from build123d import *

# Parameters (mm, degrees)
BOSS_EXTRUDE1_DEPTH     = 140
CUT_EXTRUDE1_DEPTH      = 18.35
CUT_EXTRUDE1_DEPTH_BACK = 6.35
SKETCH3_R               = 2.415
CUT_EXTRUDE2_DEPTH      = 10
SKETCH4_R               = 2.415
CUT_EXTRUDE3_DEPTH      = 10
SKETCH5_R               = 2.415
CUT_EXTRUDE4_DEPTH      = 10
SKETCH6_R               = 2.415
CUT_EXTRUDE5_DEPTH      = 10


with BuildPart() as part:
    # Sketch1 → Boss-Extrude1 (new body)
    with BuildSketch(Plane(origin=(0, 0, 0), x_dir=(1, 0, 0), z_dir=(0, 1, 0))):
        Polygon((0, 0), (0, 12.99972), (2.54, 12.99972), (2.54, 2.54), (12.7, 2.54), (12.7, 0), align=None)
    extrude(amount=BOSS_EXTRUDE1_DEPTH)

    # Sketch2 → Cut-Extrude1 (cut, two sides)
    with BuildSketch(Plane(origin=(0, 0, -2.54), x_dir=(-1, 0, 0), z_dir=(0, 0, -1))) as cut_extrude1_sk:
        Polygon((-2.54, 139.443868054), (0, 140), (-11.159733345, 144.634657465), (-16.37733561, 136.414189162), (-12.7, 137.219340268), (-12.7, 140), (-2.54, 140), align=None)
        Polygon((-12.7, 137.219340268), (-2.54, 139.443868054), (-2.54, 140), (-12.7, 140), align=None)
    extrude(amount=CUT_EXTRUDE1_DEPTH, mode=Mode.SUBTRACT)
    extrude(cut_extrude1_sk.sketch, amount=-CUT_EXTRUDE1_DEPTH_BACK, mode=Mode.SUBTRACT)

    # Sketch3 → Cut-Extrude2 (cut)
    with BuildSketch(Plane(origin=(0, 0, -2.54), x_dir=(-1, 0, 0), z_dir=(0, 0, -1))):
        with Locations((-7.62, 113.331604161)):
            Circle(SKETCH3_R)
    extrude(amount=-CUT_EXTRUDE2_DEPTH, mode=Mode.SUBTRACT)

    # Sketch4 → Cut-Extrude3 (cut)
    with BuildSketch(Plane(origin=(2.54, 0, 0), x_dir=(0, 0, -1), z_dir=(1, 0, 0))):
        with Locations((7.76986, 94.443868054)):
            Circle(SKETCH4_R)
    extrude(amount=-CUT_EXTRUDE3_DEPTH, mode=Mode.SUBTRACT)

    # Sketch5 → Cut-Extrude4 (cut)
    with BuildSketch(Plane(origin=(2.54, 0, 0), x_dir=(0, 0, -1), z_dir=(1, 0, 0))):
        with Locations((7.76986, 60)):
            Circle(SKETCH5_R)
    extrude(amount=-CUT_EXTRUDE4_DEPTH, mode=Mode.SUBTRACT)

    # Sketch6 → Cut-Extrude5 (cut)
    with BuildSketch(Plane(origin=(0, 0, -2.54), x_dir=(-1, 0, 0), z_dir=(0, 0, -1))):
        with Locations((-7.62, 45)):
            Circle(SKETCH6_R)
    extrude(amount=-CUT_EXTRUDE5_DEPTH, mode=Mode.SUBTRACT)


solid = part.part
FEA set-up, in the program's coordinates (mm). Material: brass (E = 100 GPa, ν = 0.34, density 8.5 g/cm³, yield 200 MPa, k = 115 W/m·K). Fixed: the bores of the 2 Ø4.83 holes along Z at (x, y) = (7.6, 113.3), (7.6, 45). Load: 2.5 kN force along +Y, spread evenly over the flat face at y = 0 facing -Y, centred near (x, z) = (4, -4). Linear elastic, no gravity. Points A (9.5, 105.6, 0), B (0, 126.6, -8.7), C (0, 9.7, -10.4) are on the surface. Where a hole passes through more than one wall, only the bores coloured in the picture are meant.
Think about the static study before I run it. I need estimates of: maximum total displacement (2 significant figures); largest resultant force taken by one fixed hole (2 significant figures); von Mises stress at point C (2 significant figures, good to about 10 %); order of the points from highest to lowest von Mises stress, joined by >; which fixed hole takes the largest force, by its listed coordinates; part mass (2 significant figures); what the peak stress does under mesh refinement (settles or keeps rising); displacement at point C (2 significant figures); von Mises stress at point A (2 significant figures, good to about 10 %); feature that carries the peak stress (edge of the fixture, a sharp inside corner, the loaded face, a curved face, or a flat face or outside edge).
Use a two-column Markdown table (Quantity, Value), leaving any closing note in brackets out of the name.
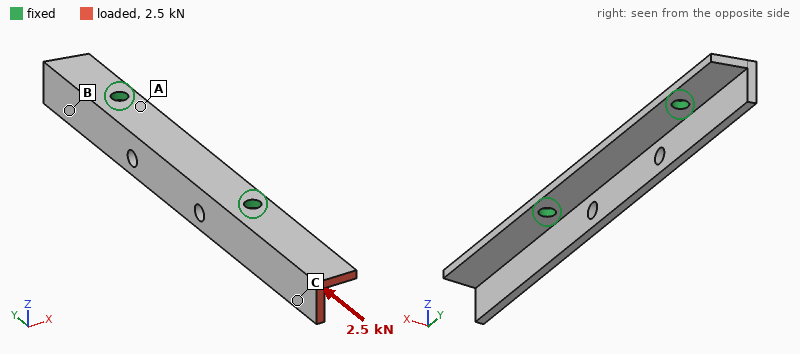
| Quantity | Value |
|---|---|
| maximum total displacement | 68 µm |
| largest resultant force taken by one fixed hole | 2.0 kN |
| von Mises stress at point C | 43 MPa |
| order of the points from highest to lowest von Mises stress, joined by > | C > A > B |
| which fixed hole takes the largest force, by its listed coordinates | (7.6, 45) |
| part mass | 68 g |
| what the peak stress does under mesh refinement | keeps rising |
| displacement at point C | 55 µm |
| von Mises stress at point A | 18 MPa |
| feature that carries the peak stress | edge of the fixture |
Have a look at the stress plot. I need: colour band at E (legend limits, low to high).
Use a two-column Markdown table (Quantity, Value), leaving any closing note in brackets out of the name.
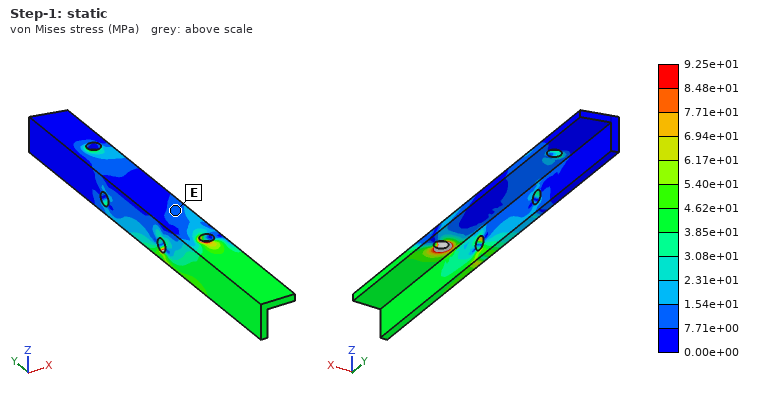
| Quantity | Value |
|---|---|
| colour band at E | 7.71e+00 to 1.54e+01 MPa |
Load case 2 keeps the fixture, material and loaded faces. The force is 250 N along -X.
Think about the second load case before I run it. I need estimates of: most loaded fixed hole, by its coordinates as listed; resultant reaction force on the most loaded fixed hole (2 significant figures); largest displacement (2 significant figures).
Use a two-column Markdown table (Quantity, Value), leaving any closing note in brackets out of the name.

| Quantity | Value |
|---|---|
| most loaded fixed hole, by its coordinates as listed | (7.6, 45) |
| resultant reaction force on the most loaded fixed hole | 340 N |
| largest displacement | 0.30 mm |
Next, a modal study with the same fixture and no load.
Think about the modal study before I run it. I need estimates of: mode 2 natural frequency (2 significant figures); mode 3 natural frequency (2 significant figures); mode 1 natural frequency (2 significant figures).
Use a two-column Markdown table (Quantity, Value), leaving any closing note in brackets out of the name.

| Quantity | Value |
|---|---|
| mode 2 natural frequency | 2300 Hz |
| mode 3 natural frequency | 3300 Hz |
| mode 1 natural frequency | 1800 Hz |
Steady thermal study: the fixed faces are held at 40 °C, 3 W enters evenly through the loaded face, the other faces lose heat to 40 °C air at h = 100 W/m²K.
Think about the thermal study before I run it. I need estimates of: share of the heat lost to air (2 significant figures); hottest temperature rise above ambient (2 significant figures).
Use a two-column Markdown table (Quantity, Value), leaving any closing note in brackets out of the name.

| Quantity | Value |
|---|---|
| share of the heat lost to air | 52 % |
| hottest temperature rise above ambient | 14 K |
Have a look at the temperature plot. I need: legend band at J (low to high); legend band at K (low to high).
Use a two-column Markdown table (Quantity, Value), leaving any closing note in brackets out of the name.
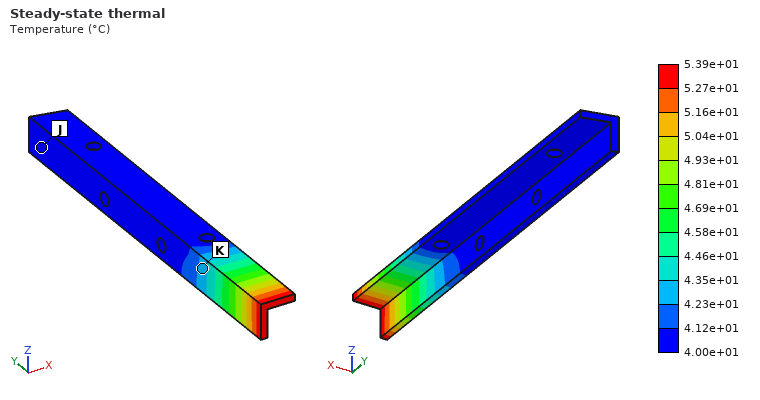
| Quantity | Value |
|---|---|
| legend band at J | 4.00e+01 to 4.12e+01 °C |
| legend band at K | 4.23e+01 to 4.35e+01 °C |
